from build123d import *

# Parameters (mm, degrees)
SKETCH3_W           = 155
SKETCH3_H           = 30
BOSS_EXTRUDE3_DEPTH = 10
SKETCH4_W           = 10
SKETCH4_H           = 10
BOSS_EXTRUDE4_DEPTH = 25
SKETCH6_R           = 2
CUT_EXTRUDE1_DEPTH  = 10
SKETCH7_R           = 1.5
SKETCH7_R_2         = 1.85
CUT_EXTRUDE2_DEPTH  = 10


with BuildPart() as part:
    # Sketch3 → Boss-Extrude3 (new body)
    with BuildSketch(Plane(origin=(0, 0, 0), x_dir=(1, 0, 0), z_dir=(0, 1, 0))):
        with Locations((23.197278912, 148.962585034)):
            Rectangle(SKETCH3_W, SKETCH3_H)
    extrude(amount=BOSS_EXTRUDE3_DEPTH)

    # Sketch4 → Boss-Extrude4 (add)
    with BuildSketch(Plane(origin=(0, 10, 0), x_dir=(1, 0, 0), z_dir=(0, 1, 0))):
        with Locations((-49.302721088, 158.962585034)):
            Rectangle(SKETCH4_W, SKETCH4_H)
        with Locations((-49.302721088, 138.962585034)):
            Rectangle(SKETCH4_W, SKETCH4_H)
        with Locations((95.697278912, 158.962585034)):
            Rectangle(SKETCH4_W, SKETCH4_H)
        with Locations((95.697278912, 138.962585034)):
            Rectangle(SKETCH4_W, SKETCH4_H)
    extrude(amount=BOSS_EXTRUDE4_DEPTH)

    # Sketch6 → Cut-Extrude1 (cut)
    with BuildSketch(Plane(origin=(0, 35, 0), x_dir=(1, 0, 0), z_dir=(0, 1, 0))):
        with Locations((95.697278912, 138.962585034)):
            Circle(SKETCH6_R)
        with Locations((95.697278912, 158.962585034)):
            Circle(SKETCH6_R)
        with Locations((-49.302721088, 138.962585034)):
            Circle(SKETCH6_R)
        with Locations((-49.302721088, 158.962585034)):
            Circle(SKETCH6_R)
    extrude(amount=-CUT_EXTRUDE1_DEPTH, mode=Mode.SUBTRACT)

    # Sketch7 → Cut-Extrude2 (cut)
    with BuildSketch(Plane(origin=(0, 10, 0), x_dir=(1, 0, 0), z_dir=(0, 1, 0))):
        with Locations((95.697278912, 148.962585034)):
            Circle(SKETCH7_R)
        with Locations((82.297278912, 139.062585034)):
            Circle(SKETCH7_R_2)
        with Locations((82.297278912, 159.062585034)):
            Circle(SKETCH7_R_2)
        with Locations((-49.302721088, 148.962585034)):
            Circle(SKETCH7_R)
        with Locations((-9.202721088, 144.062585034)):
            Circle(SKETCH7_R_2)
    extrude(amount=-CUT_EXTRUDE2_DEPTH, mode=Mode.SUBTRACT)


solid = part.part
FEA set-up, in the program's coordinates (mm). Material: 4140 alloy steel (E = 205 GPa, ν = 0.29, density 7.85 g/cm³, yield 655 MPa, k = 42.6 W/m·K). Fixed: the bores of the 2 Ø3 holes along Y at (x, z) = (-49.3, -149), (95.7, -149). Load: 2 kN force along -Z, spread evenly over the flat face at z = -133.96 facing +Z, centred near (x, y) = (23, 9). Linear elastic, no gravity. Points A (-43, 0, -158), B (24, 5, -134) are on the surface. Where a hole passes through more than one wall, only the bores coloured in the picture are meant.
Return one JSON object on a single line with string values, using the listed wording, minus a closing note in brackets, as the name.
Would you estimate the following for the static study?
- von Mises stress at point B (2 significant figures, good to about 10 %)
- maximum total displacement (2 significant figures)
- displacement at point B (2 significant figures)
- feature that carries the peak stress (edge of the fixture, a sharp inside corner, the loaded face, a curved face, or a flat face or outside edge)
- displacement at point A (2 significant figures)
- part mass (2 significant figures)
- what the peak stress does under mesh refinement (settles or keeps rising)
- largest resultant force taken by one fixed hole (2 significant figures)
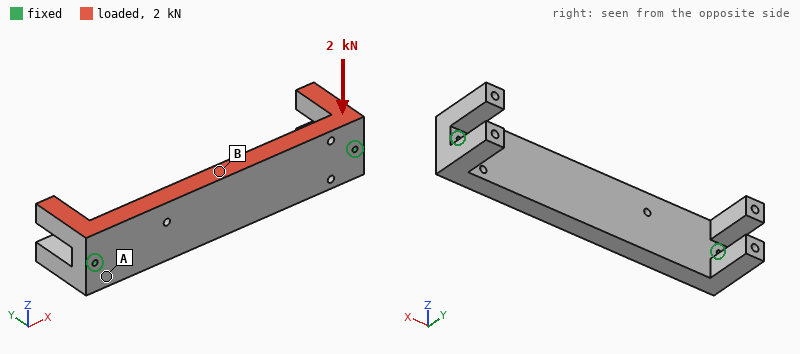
{"von Mises stress at point B": "14 MPa", "maximum total displacement": "12 µm", "displacement at point B": "11 µm", "feature that carries the peak stress": "edge of the fixture", "displacement at point A": "2.3 µm", "part mass": "440 g", "what the peak stress does under mesh refinement": "keeps rising", "largest resultant force taken by one fixed hole": "1.0 kN"}
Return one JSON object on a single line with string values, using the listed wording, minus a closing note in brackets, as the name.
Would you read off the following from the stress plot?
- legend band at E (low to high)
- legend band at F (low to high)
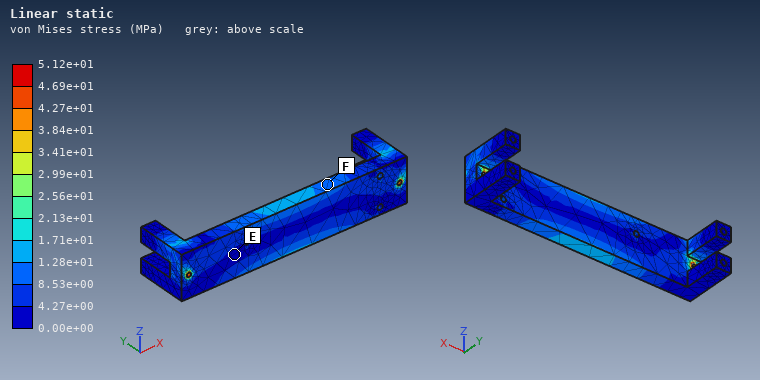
{"legend band at E": "0.00e+00 to 4.27e+00 MPa", "legend band at F": "8.53e+00 to 1.28e+01 MPa"}
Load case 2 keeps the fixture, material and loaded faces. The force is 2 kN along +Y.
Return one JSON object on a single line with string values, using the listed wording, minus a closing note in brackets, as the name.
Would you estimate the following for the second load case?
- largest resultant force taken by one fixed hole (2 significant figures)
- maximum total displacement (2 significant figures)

{"largest resultant force taken by one fixed hole": "1.0 kN", "maximum total displacement": "44 µm"}
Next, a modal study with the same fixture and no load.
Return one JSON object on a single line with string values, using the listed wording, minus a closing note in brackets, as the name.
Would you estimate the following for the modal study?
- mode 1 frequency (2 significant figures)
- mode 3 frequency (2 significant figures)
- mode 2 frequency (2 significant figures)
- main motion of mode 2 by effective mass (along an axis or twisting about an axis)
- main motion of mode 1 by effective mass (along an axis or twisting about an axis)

{"mode 1 frequency": "2100 Hz", "mode 3 frequency": "5000 Hz", "mode 2 frequency": "3400 Hz", "main motion of mode 2 by effective mass": "along Z", "main motion of mode 1 by effective mass": "along Y"}
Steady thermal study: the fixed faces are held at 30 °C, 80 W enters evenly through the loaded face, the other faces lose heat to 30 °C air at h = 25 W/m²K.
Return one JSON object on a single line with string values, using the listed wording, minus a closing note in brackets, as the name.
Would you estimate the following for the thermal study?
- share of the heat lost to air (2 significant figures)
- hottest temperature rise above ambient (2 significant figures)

{"share of the heat lost to air": "23 %", "hottest temperature rise above ambient": "84 K"}
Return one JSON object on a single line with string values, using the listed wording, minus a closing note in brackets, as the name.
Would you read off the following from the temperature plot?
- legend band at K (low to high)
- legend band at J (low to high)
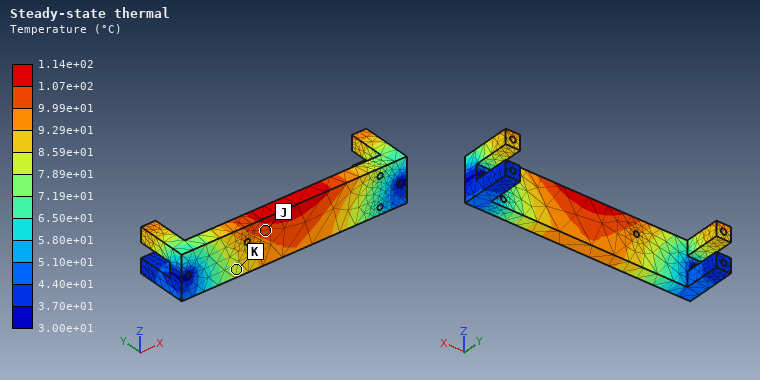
{"legend band at K": "7.89e+01 to 8.59e+01 °C", "legend band at J": "9.99e+01 to 1.07e+02 °C"}
